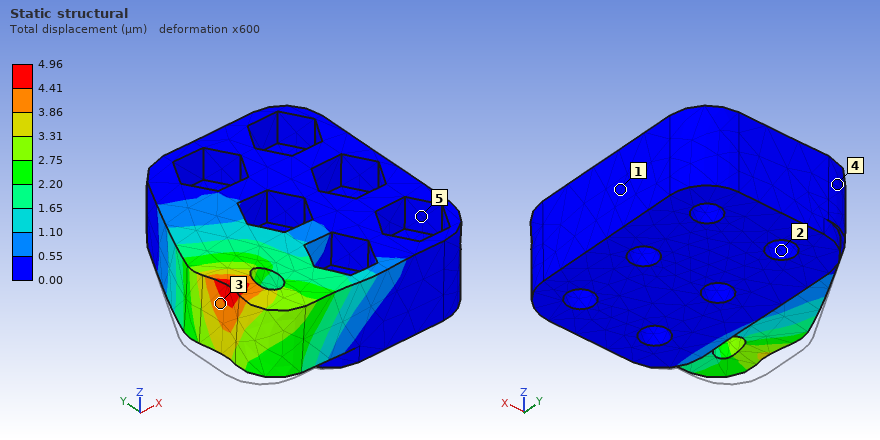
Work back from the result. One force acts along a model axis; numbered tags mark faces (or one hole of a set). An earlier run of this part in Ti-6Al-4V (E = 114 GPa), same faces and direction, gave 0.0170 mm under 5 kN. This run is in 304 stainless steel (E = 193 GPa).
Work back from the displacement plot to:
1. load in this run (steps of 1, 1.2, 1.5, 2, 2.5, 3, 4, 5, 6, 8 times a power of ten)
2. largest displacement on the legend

2.5 kN
4.96 µm
